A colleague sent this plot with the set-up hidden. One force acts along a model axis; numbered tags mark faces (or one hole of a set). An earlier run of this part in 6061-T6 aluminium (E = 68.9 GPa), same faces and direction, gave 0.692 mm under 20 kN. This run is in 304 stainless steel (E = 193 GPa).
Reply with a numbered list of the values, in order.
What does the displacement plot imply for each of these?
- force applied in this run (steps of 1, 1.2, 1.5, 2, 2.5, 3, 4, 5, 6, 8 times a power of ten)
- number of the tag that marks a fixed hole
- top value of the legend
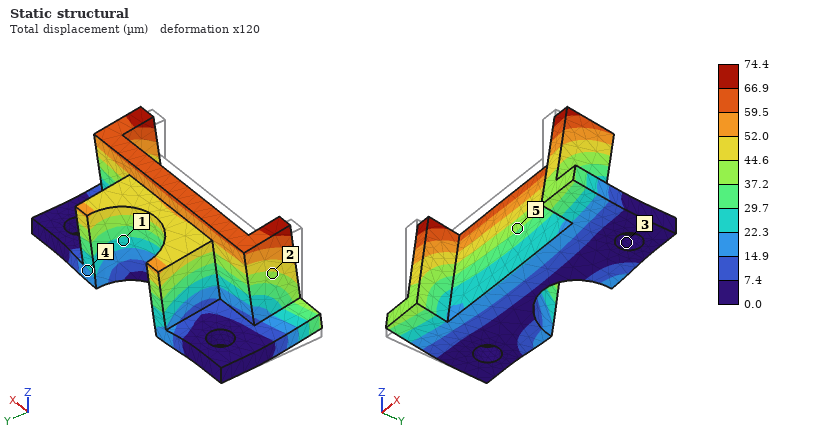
1. 6 kN
2. 3
3. 74.4 µm
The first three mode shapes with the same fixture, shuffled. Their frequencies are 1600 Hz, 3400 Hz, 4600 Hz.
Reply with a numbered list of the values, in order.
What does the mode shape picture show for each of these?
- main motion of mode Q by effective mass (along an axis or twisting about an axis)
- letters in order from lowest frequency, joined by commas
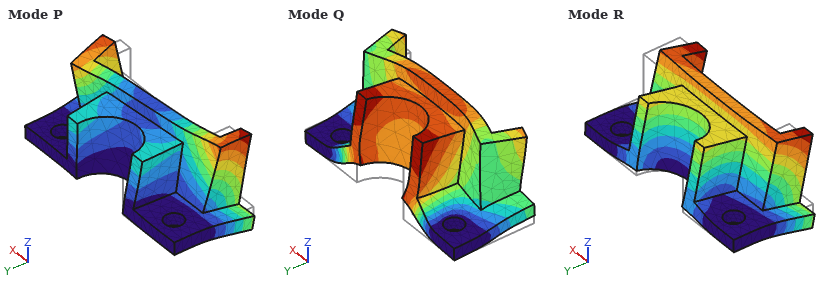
1. along Z
2. R, P, Q
